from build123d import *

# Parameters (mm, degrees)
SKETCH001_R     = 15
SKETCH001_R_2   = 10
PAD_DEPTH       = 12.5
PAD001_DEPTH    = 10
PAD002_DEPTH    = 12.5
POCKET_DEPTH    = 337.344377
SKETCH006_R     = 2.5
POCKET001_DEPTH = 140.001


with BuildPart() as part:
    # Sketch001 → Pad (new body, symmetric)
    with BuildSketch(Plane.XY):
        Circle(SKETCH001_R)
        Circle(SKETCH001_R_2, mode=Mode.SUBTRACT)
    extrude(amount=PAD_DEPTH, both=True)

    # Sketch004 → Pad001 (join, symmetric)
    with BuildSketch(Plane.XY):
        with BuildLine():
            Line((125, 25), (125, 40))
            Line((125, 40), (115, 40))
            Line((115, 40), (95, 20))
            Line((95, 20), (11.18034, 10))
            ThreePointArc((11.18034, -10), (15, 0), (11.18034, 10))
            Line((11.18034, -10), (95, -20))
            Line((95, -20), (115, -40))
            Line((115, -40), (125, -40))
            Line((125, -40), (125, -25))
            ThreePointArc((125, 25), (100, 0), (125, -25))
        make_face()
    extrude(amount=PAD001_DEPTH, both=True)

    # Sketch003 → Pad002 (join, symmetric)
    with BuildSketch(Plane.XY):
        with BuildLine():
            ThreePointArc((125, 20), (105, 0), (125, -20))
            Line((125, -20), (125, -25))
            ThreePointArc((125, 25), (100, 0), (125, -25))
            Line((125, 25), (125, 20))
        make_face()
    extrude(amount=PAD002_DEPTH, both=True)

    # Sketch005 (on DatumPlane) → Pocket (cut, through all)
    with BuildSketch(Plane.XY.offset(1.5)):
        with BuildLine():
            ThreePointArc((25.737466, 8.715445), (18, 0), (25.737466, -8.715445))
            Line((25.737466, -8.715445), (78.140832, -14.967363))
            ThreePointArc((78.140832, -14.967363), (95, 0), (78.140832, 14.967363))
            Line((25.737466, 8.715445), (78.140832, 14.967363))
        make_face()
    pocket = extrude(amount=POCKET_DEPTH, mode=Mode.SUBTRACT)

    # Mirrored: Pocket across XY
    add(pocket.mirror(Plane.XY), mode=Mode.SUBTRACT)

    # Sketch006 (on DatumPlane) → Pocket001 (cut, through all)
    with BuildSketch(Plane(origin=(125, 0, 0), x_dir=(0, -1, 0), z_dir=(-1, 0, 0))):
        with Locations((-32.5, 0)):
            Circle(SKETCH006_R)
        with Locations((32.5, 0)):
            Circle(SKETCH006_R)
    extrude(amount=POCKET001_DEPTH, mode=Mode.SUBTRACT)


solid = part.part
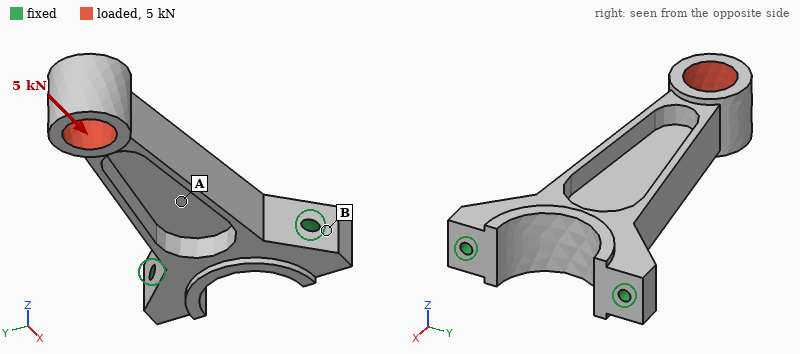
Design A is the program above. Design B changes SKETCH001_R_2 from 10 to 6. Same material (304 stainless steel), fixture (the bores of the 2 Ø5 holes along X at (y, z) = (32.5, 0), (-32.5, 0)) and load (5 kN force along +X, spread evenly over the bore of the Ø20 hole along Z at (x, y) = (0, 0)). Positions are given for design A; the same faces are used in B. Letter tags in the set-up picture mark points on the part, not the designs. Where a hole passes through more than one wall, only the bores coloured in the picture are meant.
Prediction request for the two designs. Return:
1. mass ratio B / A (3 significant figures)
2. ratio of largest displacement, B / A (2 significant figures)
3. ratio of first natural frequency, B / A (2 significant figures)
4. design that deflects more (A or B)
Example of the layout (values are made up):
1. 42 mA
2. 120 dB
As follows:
1. 1.09
2. 0.75
3. 0.85
4. A
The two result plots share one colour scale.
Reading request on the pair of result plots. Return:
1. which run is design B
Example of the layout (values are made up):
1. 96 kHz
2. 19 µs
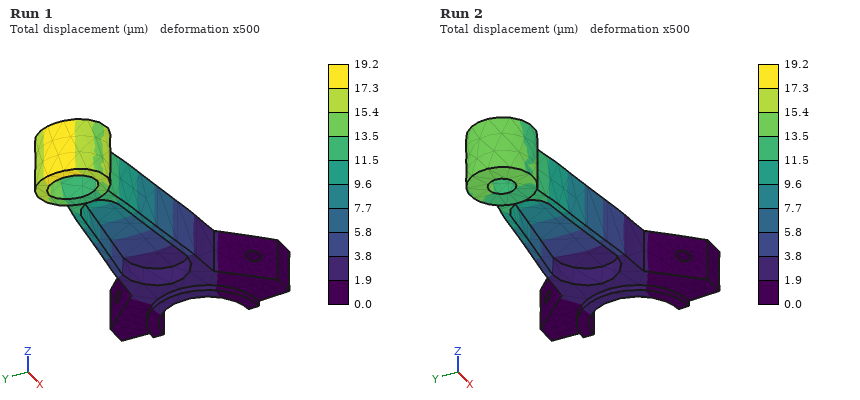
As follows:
1. Run 2
